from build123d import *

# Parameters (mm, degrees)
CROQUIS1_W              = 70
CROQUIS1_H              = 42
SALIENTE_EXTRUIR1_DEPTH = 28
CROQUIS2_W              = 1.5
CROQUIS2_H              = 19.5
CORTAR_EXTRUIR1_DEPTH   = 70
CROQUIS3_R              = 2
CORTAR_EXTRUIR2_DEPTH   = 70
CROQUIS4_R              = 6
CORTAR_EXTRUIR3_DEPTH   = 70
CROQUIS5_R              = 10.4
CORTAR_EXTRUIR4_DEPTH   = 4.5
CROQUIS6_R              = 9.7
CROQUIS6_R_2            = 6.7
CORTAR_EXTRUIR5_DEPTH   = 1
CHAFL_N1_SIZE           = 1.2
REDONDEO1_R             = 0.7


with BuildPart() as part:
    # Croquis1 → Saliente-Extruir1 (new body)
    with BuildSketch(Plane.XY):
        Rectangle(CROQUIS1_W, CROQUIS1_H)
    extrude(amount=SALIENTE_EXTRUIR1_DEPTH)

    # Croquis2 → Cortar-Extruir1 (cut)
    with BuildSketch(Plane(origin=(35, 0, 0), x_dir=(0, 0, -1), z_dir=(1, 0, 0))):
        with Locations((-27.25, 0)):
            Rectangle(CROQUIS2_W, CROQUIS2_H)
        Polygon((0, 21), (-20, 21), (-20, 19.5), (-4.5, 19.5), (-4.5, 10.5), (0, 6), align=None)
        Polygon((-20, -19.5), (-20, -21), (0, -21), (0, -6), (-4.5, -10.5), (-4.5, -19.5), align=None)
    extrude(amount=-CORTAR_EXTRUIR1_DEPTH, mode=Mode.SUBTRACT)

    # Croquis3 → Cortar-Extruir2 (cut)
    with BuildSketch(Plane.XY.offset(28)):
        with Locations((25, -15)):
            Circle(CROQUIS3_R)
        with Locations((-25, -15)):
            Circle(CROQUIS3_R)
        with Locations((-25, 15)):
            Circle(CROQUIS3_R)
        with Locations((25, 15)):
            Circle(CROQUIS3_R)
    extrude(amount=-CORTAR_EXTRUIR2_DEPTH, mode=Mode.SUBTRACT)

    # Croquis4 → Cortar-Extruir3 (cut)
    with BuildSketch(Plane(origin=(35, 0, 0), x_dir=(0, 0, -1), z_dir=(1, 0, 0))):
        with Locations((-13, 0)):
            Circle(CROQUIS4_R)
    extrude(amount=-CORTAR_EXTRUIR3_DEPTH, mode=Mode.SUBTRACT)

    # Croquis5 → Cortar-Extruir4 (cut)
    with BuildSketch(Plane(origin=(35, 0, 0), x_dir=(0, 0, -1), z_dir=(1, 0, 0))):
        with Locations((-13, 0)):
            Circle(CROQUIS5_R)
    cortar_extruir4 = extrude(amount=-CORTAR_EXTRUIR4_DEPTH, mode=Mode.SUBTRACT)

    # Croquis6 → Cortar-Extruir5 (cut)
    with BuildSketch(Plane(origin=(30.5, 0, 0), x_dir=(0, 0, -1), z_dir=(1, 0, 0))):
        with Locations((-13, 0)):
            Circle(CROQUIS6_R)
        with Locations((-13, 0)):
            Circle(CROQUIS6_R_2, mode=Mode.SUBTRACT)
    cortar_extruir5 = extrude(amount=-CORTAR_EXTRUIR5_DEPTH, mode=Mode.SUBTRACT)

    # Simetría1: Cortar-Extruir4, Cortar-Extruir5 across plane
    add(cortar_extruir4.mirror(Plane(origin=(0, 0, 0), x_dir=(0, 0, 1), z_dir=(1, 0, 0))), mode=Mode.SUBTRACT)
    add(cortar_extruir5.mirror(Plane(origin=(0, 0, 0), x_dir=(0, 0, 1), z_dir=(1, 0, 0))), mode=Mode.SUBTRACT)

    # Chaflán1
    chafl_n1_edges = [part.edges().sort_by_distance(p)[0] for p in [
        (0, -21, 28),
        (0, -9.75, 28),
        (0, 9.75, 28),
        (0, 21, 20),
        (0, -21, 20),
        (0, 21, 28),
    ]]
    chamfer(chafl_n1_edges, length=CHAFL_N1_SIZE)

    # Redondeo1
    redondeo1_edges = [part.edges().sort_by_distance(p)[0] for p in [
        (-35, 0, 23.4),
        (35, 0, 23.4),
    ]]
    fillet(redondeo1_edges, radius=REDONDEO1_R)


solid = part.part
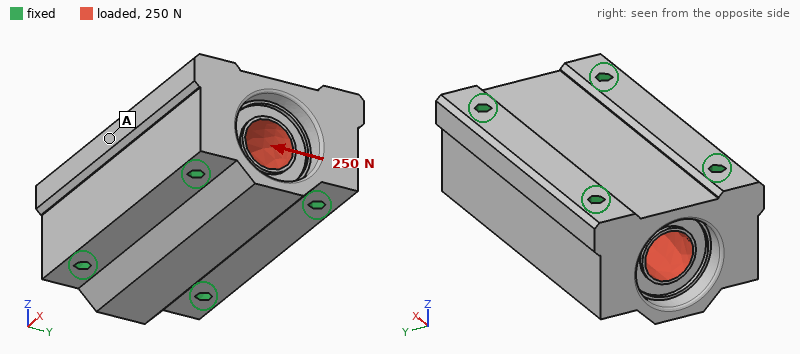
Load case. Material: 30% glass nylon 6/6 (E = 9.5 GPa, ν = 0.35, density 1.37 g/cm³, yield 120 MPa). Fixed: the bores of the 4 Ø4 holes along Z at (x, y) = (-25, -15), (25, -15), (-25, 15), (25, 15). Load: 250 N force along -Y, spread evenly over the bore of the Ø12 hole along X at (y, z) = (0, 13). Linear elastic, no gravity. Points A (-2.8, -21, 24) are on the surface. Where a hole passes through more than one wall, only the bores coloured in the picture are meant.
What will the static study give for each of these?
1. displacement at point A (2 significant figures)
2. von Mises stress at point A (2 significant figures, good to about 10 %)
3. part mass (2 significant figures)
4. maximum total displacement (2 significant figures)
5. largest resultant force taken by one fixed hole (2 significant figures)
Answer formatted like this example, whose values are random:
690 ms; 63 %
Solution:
0.55 µm; 0.13 MPa; 78 g; 0.83 µm; 68 N
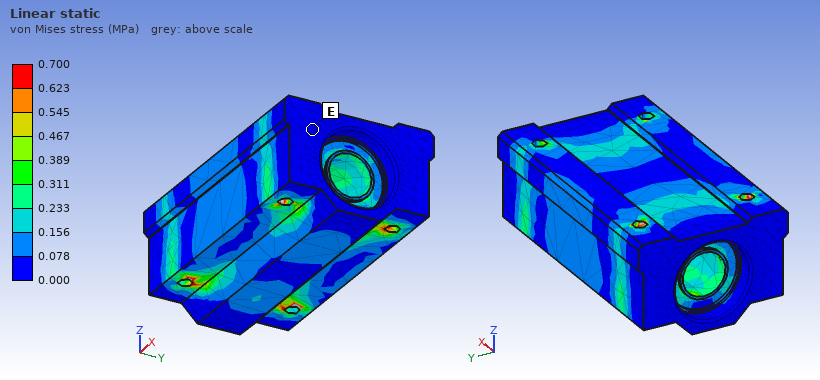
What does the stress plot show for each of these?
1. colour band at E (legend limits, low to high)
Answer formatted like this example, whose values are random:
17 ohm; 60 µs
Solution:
0.000 to 0.078 MPa
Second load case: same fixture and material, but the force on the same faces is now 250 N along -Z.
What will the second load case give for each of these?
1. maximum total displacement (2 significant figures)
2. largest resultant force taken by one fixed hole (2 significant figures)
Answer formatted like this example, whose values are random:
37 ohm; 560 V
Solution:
1.1 µm; 63 N
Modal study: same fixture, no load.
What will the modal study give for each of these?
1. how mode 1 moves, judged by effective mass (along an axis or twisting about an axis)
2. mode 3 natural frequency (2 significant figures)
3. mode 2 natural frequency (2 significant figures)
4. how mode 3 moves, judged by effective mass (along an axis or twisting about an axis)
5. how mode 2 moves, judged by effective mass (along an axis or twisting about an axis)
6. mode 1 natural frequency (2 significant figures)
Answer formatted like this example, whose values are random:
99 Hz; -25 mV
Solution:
along Z; 14 kHz; 13 kHz; twisting about X; along Y; 11 kHz
